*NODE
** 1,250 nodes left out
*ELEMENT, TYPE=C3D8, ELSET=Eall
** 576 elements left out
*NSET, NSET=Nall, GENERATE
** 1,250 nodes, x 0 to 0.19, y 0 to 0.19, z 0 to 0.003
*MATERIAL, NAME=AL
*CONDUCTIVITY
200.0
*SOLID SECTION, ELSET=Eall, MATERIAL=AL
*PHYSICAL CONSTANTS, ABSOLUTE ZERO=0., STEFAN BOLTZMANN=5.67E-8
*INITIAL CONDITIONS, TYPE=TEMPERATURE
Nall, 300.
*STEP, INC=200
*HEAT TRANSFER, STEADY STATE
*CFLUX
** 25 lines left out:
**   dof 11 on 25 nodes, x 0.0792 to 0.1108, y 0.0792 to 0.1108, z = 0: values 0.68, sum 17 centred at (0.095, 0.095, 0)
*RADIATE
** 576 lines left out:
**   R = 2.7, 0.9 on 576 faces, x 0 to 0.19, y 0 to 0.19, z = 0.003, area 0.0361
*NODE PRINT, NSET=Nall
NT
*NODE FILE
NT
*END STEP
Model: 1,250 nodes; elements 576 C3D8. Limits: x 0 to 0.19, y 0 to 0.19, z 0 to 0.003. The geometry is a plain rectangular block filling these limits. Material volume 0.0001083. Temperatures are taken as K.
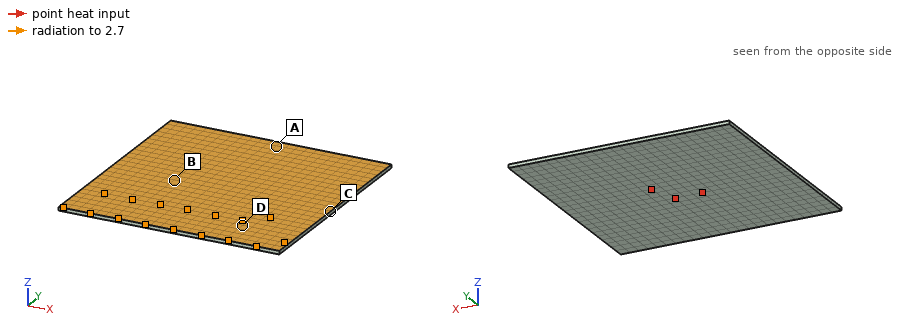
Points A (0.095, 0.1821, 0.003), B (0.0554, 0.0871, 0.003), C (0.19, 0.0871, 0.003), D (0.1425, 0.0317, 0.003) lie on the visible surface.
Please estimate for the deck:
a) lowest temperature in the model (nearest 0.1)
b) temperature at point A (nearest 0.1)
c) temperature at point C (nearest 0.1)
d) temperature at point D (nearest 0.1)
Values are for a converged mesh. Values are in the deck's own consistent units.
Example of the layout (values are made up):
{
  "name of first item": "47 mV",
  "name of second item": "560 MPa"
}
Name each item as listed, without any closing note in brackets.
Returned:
{
  "lowest temperature in the model": "308.4 K",
  "temperature at point A": "309.2 K",
  "temperature at point C": "309.2 K",
  "temperature at point D": "309.2 K"
}
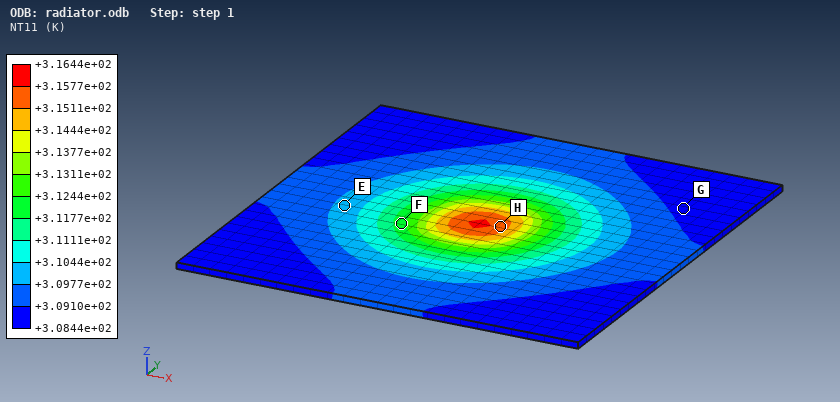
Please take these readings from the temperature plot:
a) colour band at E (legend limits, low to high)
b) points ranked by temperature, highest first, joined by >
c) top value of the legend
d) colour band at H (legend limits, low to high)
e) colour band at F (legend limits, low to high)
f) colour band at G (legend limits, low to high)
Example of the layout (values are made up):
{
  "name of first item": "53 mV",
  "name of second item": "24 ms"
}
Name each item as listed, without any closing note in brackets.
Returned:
{
  "colour band at E": "+3.0977e+02 to +3.1044e+02 K",
  "points ranked by temperature, highest first, joined by >": "H > F > E > G",
  "top value of the legend": "+3.1644e+02 K",
  "colour band at H": "+3.1511e+02 to +3.1577e+02 K",
  "colour band at F": "+3.1177e+02 to +3.1244e+02 K",
  "colour band at G": "+3.0844e+02 to +3.0910e+02 K"
}
